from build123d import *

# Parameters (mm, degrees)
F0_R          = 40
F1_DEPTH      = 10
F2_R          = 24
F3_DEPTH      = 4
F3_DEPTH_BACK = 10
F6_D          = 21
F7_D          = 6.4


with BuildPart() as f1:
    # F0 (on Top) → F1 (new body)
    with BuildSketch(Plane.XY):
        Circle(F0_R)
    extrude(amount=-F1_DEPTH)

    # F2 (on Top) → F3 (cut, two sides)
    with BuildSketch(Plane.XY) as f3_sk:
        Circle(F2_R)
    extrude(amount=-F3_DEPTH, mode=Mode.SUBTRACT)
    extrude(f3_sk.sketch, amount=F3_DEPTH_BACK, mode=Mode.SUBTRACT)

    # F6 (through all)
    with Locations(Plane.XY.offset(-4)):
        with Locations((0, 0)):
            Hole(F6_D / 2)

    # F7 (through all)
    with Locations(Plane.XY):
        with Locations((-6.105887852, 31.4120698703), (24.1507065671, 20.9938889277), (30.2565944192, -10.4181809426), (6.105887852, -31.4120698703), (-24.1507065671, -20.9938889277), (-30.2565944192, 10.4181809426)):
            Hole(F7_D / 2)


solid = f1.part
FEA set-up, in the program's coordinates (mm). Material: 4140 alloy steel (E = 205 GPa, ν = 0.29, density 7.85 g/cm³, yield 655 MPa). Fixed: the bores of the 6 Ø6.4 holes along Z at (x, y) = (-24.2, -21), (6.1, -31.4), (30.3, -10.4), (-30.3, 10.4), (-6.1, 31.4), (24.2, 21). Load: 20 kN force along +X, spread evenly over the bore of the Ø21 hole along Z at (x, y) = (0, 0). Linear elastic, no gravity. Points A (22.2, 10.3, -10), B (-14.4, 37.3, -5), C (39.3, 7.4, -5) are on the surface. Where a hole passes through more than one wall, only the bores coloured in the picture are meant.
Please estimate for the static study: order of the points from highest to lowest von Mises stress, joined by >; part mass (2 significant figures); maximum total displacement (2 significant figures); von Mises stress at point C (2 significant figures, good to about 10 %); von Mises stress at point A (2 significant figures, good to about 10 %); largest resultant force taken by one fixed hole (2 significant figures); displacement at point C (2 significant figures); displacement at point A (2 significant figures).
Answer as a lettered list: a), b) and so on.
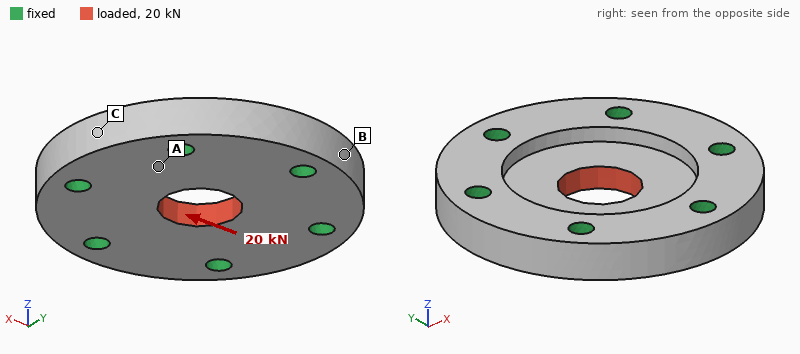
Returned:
a) A > C > B
b) 310 g
c) 5.1 µm
d) 15 MPa
e) 25 MPa
f) 4.7 kN
g) 1.5 µm
h) 2.2 µm
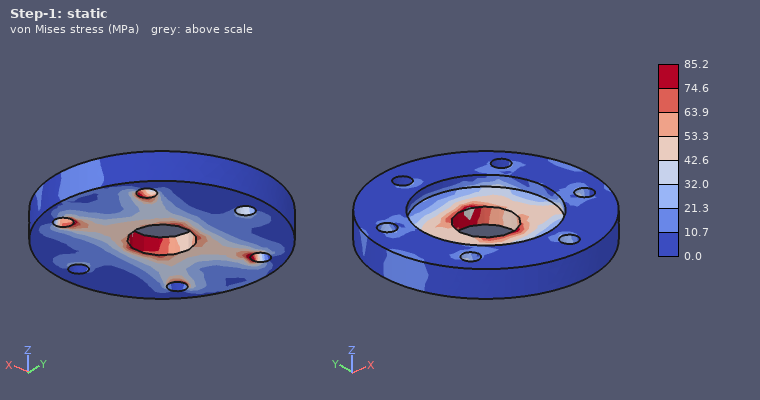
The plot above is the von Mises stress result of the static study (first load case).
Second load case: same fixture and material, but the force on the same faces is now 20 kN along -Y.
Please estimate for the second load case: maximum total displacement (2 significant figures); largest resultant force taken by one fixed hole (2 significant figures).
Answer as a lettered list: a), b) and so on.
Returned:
a) 5.1 µm
b) 4.9 kN
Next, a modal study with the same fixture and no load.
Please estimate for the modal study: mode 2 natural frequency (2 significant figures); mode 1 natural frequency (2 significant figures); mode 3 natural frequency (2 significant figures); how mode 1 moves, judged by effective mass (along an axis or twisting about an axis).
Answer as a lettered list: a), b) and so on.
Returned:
a) 27 kHz
b) 20 kHz
c) 27 kHz
d) along Z
